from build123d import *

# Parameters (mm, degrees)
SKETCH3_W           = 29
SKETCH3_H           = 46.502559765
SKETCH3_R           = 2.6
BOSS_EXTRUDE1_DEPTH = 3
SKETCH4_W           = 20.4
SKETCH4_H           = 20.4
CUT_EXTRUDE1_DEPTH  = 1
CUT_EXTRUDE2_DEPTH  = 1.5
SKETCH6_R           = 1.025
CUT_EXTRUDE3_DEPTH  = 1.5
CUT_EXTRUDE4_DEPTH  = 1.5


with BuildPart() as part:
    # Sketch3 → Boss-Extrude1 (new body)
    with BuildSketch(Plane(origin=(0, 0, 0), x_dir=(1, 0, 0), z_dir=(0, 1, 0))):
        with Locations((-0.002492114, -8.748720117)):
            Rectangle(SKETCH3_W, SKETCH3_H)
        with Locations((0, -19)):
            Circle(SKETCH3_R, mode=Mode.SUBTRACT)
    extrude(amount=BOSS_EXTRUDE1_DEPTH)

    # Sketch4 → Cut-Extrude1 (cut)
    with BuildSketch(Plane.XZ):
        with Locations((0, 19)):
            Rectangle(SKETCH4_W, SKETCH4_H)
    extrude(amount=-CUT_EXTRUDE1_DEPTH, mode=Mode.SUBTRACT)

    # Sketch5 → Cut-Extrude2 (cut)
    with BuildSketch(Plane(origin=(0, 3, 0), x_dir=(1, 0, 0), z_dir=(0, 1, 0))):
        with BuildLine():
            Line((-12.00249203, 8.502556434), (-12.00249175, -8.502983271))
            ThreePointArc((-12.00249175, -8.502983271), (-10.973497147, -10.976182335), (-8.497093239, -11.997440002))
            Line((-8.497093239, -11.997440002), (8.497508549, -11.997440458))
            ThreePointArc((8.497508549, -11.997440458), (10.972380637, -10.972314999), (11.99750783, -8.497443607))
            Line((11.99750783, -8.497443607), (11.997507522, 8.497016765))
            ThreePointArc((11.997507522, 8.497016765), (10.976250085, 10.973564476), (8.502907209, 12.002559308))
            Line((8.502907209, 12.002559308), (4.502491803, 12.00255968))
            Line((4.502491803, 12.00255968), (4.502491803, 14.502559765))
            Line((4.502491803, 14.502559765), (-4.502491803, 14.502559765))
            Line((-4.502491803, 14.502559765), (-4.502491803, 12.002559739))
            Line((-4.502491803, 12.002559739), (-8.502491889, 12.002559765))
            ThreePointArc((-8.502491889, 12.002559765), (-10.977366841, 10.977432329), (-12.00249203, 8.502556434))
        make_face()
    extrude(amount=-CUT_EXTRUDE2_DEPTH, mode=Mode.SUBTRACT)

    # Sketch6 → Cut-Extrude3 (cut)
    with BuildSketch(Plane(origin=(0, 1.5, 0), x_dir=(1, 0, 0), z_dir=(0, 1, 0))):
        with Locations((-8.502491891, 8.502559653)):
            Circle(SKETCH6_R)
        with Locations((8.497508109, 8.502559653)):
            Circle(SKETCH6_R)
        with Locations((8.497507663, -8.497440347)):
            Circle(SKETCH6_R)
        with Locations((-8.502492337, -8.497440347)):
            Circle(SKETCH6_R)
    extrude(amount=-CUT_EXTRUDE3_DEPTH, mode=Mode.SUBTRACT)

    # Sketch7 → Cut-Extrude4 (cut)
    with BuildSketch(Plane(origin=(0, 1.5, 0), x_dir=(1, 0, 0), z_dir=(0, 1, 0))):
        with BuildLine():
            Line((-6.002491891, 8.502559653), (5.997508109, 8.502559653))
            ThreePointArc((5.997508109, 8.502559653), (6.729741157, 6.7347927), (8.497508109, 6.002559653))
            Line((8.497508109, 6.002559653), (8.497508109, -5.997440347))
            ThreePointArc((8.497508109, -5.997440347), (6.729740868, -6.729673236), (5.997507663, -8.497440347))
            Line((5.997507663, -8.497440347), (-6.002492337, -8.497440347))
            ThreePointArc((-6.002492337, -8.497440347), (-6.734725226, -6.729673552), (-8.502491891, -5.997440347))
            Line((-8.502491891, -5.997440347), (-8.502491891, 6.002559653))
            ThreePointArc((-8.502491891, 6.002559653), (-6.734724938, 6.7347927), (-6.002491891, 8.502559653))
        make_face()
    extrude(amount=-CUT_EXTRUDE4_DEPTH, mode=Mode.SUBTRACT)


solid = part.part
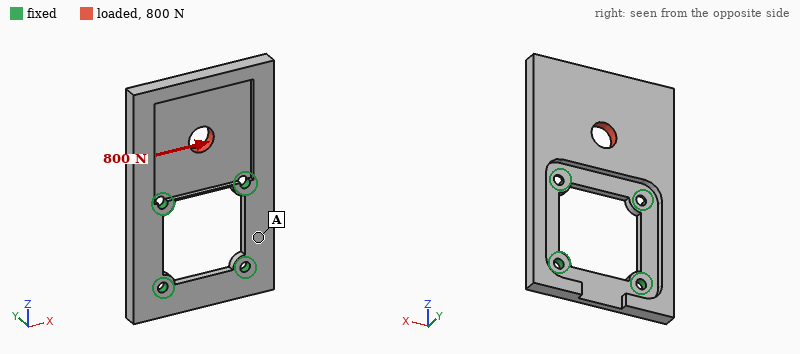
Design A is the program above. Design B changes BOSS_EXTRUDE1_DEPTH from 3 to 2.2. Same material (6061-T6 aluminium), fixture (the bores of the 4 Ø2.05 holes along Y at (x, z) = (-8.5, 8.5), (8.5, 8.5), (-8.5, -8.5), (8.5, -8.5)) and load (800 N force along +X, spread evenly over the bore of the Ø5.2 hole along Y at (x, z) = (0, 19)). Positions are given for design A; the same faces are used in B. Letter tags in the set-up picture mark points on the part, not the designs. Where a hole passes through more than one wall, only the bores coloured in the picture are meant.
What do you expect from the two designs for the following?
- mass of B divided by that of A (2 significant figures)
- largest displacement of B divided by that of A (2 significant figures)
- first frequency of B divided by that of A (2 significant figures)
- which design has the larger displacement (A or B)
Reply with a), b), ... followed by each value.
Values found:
a) 0.74
b) 1.4
c) 0.87
d) B
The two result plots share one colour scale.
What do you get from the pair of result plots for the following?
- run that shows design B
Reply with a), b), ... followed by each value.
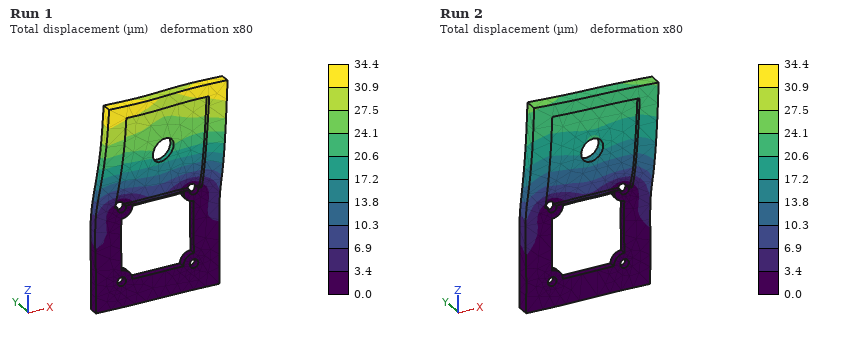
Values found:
a) Run 1
